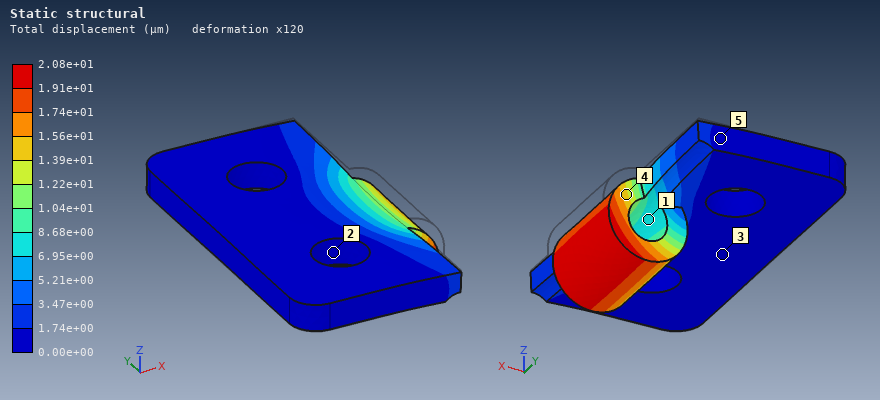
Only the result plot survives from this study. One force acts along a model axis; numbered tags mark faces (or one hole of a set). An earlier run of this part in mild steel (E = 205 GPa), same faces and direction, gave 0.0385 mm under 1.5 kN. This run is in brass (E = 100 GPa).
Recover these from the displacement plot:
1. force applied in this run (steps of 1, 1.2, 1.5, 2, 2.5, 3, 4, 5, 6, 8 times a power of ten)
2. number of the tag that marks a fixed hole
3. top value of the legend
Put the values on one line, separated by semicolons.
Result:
400 N; 2; 2.08e+01 µm
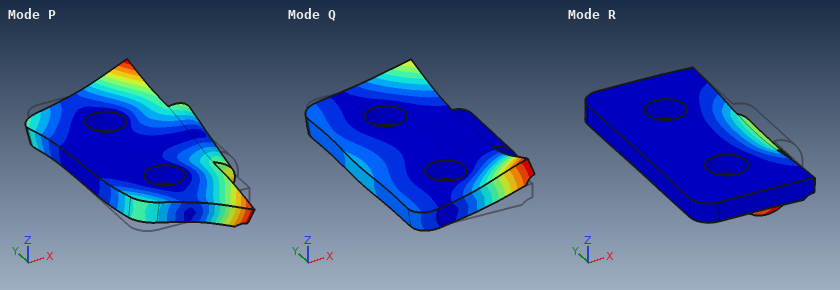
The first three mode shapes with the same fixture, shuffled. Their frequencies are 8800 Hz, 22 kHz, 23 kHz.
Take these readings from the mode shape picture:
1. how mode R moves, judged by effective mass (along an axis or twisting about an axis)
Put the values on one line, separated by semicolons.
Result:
along Z
